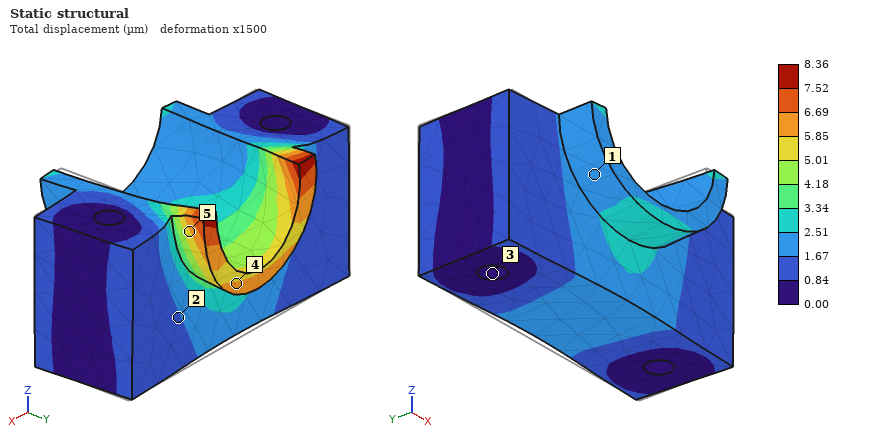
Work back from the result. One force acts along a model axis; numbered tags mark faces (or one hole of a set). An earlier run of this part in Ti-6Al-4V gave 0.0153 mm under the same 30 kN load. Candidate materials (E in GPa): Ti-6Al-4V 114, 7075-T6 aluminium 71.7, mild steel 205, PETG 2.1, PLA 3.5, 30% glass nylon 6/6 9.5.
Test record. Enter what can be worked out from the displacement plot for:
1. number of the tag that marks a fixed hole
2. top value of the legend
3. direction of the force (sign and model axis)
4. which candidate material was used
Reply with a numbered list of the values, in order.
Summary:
1. 3
2. 8.36 µm
3. -Y
4. mild steel
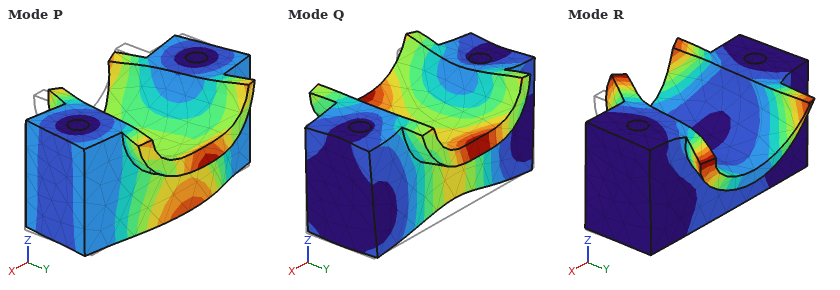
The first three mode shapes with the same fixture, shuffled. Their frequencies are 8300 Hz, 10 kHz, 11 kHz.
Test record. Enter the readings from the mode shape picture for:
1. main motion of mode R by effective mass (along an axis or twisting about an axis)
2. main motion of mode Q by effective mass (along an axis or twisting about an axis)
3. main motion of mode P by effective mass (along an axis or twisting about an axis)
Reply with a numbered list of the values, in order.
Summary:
1. twisting about X
2. along Z
3. along Y
